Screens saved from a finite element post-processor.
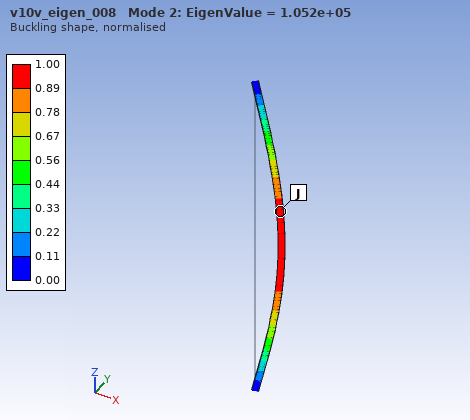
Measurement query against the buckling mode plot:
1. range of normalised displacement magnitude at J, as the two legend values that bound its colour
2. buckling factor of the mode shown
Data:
0.89 to 1.00
1.052e+05
